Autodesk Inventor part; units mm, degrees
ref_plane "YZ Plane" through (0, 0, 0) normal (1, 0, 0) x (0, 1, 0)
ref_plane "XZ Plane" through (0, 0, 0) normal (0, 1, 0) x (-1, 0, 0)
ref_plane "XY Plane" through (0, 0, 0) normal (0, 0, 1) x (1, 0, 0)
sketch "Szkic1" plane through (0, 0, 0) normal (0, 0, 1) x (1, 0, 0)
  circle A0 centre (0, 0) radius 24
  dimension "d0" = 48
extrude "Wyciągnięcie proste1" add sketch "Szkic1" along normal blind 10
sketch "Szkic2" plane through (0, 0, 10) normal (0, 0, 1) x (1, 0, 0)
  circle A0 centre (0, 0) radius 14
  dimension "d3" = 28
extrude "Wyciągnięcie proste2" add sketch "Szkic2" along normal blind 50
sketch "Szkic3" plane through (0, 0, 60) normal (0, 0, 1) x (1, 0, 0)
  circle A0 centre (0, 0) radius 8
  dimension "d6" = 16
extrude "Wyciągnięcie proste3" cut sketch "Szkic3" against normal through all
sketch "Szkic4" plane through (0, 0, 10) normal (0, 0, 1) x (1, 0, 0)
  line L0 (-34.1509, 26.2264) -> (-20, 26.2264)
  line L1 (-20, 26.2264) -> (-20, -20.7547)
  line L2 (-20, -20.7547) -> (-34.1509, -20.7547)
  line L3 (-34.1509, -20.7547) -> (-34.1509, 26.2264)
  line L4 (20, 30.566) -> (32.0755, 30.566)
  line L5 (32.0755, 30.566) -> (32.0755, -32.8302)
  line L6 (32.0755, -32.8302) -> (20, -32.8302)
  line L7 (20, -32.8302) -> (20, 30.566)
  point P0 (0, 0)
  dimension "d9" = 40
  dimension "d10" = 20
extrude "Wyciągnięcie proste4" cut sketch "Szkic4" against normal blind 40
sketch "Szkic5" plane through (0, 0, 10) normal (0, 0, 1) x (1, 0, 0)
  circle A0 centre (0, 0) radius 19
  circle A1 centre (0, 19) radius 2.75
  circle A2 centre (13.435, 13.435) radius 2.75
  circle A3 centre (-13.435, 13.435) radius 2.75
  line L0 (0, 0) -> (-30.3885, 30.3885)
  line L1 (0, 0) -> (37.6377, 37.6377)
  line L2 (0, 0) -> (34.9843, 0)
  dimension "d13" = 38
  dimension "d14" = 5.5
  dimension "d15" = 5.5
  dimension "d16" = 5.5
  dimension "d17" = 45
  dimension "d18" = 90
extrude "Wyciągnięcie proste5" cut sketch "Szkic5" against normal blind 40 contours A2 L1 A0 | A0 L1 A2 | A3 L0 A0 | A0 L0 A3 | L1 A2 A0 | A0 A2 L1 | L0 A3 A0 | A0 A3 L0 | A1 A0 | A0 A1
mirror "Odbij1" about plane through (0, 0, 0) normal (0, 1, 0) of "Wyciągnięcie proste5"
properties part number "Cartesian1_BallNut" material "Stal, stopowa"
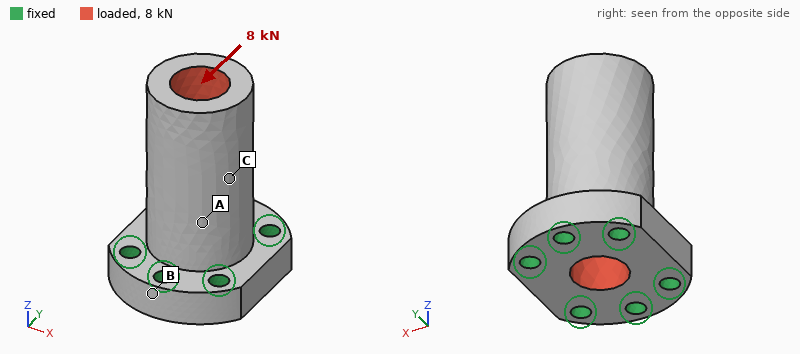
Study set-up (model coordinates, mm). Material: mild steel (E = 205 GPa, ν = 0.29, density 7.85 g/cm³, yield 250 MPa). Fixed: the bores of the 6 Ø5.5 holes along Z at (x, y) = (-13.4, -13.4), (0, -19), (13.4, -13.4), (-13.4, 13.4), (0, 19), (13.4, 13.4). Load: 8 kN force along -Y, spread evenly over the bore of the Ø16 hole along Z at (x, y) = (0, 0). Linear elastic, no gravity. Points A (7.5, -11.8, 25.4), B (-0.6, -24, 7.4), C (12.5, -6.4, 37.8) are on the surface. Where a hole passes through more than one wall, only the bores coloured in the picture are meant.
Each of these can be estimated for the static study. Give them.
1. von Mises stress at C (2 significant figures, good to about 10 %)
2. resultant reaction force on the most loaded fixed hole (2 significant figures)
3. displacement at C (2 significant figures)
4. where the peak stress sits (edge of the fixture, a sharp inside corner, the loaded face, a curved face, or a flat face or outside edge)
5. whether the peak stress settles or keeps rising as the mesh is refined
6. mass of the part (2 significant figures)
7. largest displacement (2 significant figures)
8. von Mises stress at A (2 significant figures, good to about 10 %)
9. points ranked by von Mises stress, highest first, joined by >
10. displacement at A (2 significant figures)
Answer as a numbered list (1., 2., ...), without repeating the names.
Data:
1. 19 MPa
2. 3.5 kN
3. 21 µm
4. a sharp inside corner
5. keeps rising
6. 270 g
7. 39 µm
8. 36 MPa
9. A > C > B
10. 13 µm
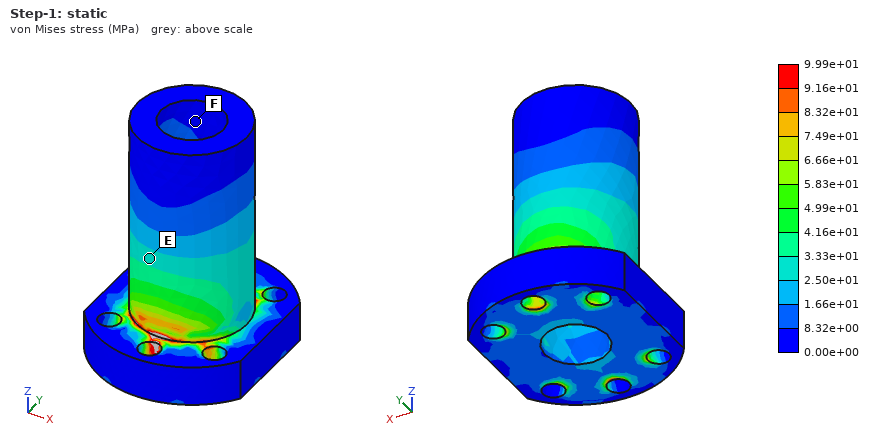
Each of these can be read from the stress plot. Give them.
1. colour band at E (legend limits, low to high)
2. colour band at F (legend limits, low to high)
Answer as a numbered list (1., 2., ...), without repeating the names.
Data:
1. 2.50e+01 to 3.33e+01 MPa
2. 0.00e+00 to 8.32e+00 MPa
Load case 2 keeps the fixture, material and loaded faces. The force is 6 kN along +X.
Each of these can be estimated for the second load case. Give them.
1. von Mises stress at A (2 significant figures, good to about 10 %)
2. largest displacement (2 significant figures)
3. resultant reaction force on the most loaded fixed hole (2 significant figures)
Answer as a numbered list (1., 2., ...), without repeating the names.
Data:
1. 24 MPa
2. 33 µm
3. 3.1 kN
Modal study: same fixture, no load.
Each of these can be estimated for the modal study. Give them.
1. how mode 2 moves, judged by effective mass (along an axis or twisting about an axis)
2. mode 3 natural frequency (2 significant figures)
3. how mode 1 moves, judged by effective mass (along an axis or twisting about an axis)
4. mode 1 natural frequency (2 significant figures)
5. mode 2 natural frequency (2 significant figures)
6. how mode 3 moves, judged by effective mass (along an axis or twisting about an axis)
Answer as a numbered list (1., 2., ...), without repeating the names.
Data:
1. along Y
2. 15 kHz
3. along X
4. 5800 Hz
5. 6200 Hz
6. twisting about Z
